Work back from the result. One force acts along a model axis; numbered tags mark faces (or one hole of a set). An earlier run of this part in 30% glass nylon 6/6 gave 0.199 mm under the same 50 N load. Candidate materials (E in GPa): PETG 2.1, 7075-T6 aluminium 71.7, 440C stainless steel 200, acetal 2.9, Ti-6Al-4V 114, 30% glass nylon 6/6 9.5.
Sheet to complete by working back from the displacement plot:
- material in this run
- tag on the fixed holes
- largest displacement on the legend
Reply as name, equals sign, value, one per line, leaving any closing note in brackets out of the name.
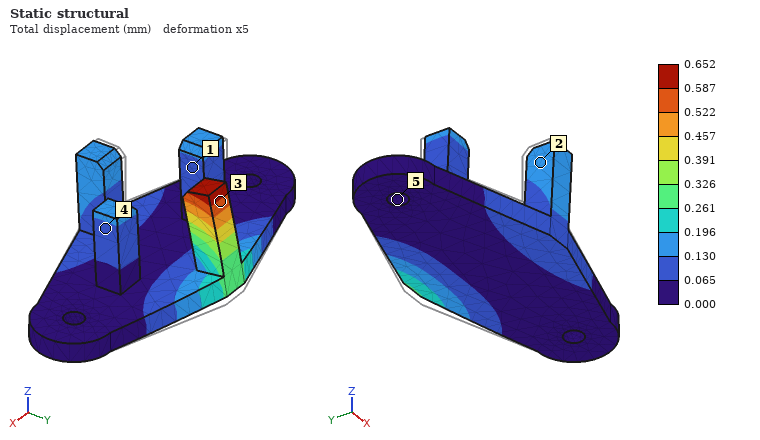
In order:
material in this run = acetal
tag on the fixed holes = 5
largest displacement on the legend = 0.652 mm
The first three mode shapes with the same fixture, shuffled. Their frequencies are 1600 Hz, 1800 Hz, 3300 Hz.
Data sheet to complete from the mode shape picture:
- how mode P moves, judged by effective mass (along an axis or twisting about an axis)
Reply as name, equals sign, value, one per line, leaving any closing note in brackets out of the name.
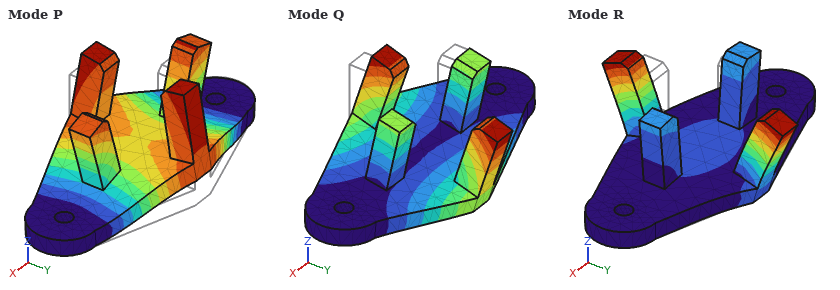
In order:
how mode P moves, judged by effective mass = along Z
